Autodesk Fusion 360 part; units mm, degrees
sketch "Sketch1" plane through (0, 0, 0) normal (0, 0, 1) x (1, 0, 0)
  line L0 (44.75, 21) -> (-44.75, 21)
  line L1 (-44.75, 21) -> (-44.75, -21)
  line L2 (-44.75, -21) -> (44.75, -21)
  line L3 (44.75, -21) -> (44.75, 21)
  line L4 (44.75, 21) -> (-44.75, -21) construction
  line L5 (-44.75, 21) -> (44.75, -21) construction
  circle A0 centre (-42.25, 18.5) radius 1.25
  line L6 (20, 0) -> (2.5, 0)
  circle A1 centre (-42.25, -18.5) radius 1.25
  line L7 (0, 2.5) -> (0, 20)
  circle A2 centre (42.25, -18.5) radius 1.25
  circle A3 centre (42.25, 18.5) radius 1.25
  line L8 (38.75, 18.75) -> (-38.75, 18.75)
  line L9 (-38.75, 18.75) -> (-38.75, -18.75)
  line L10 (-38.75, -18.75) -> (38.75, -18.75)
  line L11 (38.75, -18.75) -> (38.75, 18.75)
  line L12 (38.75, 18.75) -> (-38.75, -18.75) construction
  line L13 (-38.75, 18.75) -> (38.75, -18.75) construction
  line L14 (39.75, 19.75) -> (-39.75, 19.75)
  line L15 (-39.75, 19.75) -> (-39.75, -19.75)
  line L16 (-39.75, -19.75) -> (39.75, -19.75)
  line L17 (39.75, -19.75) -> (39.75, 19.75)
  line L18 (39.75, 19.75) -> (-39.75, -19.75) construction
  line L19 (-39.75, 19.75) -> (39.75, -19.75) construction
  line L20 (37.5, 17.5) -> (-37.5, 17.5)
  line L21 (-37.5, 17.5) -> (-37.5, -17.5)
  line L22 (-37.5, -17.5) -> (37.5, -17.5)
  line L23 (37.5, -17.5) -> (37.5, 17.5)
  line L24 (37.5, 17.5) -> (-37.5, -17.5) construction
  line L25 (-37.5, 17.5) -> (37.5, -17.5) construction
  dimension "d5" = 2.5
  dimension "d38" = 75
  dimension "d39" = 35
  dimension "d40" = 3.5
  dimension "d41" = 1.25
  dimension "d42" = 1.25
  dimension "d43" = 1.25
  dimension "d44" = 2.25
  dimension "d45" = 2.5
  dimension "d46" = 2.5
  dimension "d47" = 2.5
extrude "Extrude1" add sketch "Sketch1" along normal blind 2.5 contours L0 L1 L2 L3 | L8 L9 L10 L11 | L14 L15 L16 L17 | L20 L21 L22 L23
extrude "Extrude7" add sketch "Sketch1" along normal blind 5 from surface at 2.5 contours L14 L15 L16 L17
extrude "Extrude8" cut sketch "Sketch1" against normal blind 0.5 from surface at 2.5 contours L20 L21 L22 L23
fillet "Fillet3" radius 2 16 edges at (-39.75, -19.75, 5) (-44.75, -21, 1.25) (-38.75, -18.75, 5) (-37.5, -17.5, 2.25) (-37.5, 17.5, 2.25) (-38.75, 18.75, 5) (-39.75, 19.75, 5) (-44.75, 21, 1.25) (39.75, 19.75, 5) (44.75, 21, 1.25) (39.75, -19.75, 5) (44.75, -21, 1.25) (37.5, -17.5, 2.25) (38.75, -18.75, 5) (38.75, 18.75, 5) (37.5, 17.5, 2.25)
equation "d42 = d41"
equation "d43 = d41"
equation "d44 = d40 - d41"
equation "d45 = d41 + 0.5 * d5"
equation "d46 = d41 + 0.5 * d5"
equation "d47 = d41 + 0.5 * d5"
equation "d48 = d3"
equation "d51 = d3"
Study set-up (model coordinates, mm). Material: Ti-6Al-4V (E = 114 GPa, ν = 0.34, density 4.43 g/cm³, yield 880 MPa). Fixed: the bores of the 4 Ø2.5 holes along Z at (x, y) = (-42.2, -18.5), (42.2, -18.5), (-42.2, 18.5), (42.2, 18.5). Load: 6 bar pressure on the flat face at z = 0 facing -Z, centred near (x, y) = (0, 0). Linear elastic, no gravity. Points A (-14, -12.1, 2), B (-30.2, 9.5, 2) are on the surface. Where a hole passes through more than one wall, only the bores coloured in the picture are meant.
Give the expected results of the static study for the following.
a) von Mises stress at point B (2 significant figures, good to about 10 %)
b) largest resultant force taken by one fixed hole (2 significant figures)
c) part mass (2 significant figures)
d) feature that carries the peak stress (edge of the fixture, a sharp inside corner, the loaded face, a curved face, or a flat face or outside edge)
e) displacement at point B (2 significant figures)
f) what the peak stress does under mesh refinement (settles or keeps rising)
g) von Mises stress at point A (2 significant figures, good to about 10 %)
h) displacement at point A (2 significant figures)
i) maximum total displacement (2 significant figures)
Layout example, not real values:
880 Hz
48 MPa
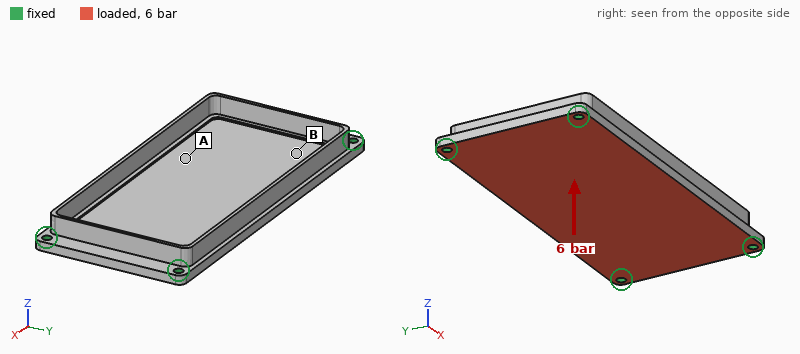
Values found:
33 MPa
600 N
41 g
edge of the fixture
0.15 mm
keeps rising
64 MPa
0.33 mm
0.44 mm
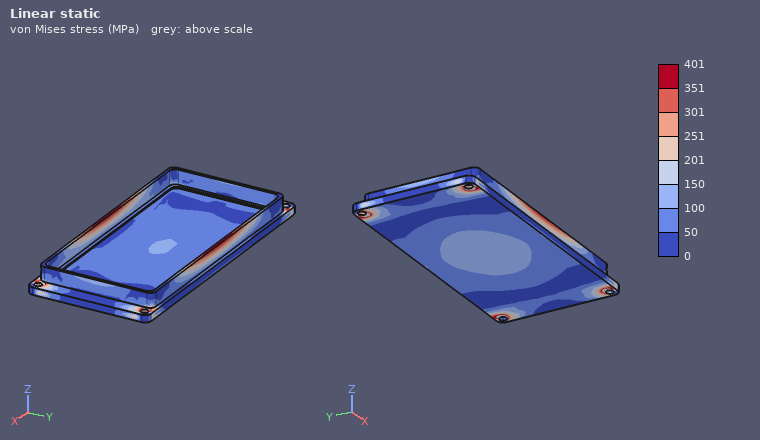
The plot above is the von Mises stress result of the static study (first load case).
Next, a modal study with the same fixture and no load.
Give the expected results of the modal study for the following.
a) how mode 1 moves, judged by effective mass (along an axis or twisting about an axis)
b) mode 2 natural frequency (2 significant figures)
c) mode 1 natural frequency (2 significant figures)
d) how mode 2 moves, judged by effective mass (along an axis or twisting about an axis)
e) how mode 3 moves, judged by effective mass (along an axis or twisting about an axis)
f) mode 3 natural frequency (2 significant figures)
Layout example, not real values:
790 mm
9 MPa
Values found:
along Z
3400 Hz
2200 Hz
twisting about X
twisting about Y
5700 Hz
